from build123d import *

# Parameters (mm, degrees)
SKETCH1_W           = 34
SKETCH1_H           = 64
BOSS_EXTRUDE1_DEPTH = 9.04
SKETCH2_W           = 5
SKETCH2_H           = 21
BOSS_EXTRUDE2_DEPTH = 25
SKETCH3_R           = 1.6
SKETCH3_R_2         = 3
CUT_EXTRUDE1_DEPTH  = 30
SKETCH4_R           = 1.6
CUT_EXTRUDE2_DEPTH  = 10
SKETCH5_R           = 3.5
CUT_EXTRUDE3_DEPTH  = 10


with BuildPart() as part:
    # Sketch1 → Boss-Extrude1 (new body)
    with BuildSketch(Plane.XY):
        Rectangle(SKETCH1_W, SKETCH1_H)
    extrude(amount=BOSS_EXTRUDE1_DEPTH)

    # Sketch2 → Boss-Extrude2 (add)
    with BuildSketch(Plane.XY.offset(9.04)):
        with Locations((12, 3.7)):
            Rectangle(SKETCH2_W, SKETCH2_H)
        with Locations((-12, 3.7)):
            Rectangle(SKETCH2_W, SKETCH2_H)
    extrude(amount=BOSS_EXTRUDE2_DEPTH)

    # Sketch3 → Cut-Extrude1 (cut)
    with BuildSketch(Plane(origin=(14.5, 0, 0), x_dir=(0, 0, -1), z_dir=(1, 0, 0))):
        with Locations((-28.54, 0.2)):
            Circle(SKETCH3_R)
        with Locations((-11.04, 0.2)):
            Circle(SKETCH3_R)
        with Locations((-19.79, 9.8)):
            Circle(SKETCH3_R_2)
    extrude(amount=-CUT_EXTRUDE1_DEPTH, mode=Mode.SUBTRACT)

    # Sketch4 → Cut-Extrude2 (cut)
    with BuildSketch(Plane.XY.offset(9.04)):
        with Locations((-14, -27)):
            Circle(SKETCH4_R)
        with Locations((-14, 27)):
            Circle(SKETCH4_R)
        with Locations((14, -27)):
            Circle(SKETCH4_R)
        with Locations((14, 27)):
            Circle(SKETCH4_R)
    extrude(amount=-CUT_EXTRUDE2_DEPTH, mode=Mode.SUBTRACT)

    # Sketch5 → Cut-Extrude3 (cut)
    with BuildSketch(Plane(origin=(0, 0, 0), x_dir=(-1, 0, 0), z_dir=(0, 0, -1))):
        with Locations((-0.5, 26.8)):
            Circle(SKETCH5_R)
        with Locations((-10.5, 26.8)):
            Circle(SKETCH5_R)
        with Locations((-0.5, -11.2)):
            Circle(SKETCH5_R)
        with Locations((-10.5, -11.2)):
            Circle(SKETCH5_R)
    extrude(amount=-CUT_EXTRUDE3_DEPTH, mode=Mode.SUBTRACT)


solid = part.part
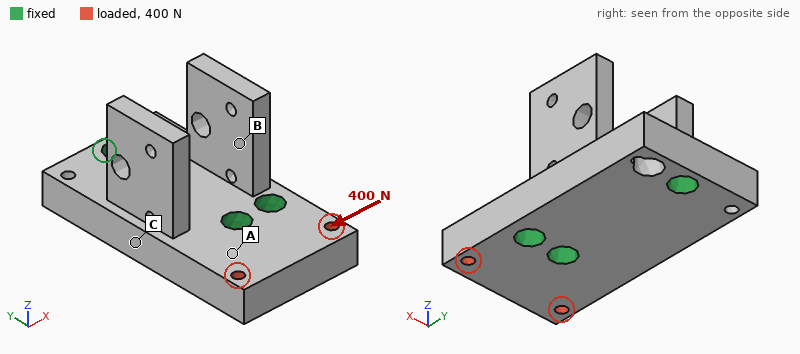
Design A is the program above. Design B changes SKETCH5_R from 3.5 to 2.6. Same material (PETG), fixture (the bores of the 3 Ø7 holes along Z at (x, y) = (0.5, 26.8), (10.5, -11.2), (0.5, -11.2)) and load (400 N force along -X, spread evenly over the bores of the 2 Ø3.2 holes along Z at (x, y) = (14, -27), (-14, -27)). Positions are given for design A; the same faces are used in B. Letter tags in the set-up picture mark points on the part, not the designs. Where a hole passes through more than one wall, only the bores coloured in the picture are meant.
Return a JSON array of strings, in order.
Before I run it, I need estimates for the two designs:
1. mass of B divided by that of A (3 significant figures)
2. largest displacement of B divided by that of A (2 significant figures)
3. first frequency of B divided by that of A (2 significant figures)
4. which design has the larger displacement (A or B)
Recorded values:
["1.03", "1.1", "0.99", "B"]
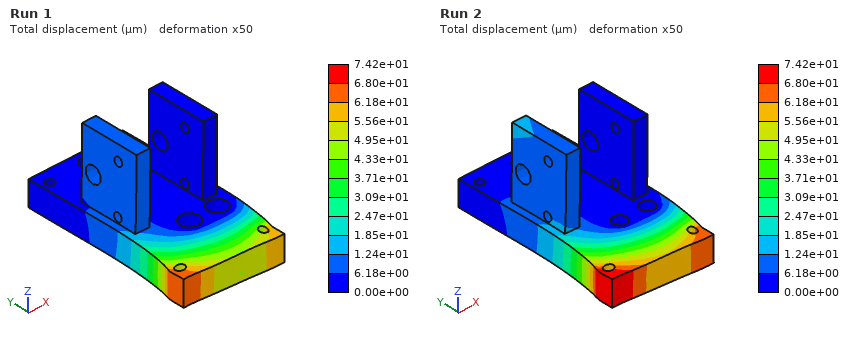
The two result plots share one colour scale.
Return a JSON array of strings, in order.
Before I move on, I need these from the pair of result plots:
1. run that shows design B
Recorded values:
["Run 2"]
